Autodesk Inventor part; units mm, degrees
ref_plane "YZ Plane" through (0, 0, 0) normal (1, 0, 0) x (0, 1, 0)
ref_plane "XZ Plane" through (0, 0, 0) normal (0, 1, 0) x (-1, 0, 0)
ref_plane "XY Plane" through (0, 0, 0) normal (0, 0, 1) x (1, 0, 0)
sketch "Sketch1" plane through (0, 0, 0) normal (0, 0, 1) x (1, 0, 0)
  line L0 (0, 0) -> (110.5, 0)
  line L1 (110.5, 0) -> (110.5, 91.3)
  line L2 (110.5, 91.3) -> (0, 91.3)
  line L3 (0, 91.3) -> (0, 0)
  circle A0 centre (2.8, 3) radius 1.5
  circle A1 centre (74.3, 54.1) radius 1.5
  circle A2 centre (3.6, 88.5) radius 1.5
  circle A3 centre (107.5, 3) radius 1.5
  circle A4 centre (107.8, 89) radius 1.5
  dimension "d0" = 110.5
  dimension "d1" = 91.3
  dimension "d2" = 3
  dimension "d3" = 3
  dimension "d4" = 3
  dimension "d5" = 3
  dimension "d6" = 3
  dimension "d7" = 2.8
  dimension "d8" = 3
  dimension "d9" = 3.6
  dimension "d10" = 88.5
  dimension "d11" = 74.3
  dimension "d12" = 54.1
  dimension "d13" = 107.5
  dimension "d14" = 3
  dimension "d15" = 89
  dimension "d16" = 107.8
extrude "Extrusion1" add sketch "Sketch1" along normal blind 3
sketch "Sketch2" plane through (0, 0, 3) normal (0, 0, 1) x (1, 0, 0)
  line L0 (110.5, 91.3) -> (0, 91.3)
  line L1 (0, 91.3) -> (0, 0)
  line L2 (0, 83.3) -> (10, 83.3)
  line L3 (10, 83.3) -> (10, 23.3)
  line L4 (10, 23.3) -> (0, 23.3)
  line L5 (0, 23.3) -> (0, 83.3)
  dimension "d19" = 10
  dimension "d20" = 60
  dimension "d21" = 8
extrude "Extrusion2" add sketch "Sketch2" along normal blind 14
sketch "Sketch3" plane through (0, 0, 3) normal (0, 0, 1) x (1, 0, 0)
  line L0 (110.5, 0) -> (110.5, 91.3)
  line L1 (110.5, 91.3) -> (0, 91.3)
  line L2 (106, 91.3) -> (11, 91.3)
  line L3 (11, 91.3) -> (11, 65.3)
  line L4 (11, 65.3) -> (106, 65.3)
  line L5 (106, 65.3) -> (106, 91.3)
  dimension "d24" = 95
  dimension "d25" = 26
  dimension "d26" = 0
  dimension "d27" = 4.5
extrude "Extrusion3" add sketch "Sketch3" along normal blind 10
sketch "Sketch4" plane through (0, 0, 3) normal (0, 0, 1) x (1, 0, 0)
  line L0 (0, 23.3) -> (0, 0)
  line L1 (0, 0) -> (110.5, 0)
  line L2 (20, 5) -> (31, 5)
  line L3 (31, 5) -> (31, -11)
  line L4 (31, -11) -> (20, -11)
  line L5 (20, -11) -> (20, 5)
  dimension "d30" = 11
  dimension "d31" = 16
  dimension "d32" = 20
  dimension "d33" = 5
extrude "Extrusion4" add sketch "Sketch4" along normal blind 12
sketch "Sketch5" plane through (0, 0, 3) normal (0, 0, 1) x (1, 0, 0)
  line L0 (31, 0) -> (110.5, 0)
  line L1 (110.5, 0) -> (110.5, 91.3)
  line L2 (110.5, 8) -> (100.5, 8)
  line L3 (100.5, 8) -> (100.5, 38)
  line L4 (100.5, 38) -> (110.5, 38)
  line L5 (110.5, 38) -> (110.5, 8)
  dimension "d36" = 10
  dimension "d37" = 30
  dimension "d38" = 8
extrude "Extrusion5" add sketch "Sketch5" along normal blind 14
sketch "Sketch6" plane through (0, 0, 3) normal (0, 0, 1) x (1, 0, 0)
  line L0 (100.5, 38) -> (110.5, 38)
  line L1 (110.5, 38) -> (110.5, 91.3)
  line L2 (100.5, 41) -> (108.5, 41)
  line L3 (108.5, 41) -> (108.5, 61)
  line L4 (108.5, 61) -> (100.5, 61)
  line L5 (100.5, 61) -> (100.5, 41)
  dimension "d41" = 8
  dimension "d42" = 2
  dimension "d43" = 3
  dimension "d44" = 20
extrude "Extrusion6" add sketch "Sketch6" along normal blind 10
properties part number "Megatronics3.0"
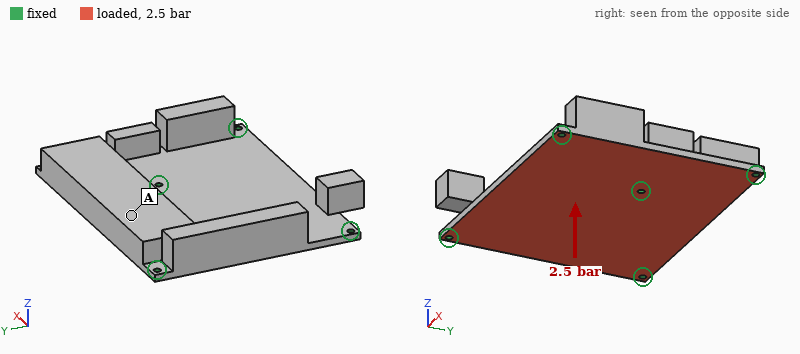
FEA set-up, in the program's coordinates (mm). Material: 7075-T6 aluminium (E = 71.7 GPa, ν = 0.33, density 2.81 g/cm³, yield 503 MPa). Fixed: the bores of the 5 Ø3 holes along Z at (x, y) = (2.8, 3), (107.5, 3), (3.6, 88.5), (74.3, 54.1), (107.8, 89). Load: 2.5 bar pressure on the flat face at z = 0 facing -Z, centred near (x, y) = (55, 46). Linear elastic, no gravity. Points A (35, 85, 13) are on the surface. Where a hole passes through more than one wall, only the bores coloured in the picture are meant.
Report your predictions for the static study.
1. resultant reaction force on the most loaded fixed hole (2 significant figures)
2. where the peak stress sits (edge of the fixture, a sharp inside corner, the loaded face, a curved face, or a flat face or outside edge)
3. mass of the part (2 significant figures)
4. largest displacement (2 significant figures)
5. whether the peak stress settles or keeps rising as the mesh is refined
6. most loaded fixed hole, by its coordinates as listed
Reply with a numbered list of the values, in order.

1. 1.2 kN
2. edge of the fixture
3. 200 g
4. 0.41 mm
5. keeps rising
6. (74.3, 54.1)
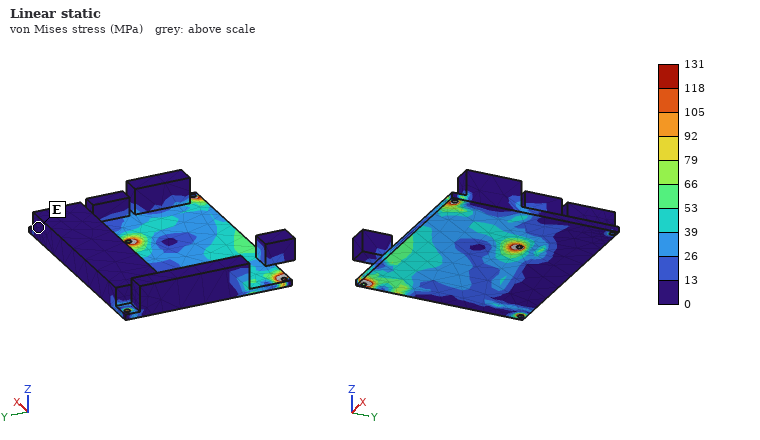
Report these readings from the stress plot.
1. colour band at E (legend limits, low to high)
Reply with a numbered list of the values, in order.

1. 0 to 13 MPa
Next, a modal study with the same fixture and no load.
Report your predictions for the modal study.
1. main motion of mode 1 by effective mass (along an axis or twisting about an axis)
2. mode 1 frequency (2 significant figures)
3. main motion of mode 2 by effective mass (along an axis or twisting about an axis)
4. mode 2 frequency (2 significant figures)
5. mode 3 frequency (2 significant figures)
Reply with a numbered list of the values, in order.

1. along Z
2. 1500 Hz
3. along Z
4. 2500 Hz
5. 2900 Hz
